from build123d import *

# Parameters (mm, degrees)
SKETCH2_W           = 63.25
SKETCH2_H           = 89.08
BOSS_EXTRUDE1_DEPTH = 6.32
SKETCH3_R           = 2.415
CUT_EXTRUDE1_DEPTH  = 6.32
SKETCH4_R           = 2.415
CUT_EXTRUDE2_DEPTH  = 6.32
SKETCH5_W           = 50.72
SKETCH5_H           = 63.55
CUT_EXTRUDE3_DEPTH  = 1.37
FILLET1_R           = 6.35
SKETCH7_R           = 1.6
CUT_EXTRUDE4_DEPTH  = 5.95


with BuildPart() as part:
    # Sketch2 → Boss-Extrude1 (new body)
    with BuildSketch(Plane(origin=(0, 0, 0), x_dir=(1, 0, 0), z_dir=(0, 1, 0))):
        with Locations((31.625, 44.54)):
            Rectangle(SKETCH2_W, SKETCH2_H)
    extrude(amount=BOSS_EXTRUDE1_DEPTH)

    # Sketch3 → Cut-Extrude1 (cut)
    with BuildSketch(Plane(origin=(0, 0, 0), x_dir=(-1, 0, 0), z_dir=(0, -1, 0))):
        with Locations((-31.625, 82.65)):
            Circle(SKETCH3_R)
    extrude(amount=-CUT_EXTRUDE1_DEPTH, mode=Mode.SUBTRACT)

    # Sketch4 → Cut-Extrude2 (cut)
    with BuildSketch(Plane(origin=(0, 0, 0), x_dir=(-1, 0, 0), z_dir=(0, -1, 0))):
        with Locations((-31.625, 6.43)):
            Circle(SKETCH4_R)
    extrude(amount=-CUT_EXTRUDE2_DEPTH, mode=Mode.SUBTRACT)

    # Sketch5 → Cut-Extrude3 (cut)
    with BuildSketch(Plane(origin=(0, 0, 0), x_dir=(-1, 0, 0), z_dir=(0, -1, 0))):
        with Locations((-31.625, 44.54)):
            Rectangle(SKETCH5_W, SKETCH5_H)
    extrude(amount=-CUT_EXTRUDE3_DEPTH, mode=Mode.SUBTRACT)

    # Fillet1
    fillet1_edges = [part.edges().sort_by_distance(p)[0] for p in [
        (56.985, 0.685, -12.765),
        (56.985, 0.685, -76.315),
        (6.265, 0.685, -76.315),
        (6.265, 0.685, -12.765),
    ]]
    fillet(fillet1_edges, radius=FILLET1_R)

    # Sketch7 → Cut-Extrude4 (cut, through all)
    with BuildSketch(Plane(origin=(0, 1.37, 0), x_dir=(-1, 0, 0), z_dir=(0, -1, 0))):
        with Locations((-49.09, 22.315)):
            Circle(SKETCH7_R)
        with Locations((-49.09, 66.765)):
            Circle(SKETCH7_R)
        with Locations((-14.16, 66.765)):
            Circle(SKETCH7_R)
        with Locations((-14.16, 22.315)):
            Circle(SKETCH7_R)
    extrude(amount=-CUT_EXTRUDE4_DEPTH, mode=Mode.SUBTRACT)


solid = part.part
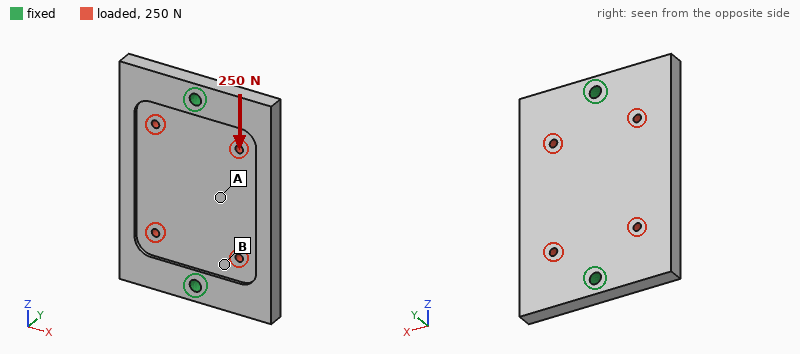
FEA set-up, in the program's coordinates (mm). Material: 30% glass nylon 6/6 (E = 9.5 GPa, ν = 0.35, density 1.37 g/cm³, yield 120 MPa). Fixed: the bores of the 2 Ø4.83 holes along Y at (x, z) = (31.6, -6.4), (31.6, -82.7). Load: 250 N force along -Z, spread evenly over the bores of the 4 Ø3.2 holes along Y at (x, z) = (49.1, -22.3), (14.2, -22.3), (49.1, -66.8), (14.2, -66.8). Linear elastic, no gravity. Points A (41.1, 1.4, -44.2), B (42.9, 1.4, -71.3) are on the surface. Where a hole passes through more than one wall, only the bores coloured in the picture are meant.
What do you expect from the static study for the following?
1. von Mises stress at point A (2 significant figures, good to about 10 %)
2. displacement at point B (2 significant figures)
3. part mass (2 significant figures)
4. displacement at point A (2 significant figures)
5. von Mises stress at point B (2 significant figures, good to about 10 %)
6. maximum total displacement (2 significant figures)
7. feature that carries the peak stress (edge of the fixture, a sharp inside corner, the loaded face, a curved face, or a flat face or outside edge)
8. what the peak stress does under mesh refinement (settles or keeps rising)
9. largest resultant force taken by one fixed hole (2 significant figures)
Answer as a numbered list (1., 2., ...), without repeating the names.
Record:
1. 0.26 MPa
2. 2.2 µm
3. 42 g
4. 2.6 µm
5. 0.89 MPa
6. 3.5 µm
7. edge of the fixture
8. keeps rising
9. 130 N
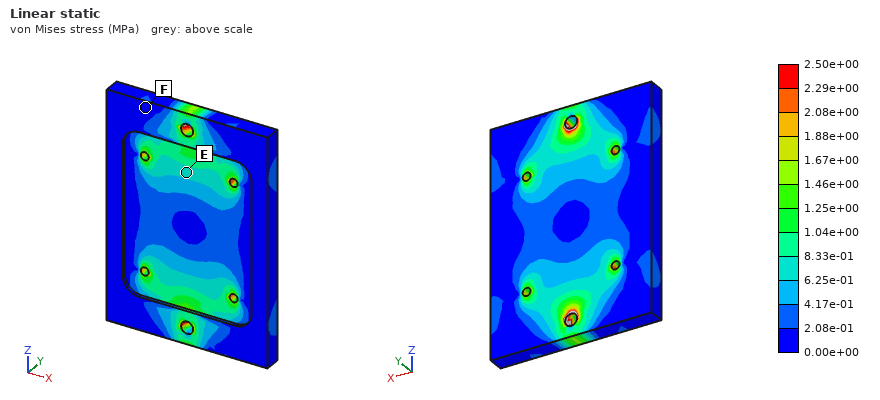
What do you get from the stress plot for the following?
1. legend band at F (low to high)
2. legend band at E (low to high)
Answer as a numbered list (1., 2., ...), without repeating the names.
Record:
1. 0.00e+00 to 2.08e-01 MPa
2. 6.25e-01 to 8.33e-01 MPa
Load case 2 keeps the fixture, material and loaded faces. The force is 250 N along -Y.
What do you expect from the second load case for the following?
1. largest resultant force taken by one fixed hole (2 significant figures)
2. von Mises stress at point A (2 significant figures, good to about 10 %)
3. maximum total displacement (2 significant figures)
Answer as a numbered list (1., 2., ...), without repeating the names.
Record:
1. 130 N
2. 2.3 MPa
3. 85 µm
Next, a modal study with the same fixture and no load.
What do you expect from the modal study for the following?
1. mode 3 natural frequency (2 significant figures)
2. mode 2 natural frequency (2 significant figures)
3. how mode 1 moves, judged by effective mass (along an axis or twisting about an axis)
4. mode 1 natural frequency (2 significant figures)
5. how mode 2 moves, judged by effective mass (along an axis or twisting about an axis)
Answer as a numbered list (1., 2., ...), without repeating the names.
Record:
1. 2800 Hz
2. 1700 Hz
3. twisting about Z
4. 1400 Hz
5. along Y
